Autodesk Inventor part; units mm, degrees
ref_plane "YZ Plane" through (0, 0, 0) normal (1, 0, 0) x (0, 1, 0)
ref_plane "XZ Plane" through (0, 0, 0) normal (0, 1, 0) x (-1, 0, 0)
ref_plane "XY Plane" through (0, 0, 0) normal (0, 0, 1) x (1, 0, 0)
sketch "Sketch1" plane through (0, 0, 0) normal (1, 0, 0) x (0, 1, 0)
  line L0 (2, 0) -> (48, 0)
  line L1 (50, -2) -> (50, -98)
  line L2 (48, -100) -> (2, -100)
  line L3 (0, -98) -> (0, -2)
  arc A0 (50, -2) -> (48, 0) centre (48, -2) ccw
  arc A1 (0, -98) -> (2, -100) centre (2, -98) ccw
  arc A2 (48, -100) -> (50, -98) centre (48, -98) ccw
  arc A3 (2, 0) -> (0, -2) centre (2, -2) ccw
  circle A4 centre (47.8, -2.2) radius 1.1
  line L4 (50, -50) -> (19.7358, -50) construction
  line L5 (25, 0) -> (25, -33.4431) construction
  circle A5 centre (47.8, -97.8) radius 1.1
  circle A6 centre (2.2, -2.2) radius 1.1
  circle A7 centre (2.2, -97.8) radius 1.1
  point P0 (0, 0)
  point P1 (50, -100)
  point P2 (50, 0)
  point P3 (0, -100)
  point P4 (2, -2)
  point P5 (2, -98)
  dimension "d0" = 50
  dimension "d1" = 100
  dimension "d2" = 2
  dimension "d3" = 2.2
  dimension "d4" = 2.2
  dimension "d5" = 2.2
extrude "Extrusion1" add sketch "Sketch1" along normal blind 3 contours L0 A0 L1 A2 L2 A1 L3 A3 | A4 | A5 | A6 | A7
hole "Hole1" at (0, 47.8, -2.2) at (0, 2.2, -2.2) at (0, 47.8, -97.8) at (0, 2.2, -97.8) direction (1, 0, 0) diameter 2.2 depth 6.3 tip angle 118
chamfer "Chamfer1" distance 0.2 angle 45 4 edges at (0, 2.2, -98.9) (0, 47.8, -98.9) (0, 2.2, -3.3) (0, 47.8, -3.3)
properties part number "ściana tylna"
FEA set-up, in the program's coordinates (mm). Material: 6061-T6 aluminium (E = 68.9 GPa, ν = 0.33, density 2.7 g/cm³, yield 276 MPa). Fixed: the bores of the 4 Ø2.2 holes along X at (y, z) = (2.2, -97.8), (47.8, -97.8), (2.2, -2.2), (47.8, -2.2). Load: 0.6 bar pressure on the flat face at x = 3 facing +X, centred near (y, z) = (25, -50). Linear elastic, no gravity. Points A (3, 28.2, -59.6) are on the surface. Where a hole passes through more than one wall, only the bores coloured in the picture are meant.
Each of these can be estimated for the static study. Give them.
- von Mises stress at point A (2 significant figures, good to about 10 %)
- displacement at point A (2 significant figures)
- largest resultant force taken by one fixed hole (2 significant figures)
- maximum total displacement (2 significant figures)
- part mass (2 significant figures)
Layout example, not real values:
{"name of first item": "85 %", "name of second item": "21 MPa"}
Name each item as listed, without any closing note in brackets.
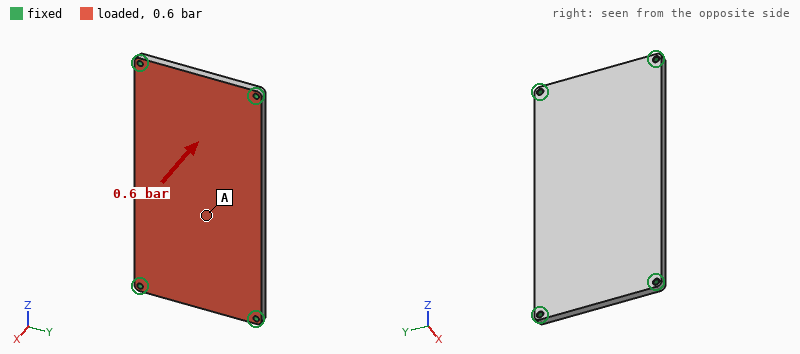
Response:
{"von Mises stress at point A": "16 MPa", "displacement at point A": "0.13 mm", "largest resultant force taken by one fixed hole": "75 N", "maximum total displacement": "0.14 mm", "part mass": "40 g"}
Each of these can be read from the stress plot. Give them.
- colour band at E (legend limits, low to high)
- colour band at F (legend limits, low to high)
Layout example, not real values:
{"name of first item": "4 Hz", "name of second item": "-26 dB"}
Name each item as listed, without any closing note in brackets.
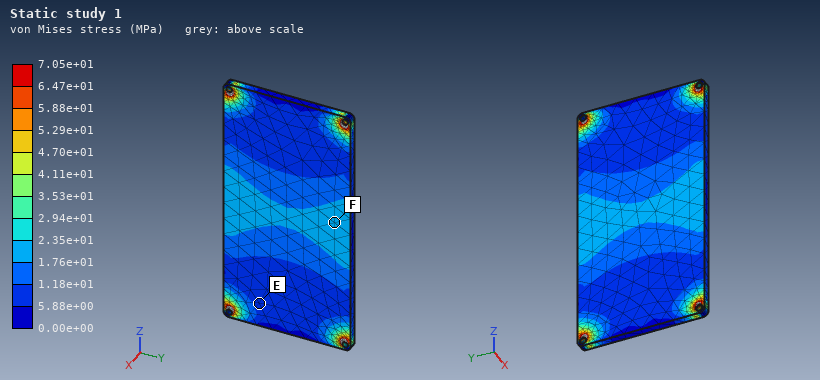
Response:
{"colour band at E": "5.88e+00 to 1.18e+01 MPa", "colour band at F": "1.76e+01 to 2.35e+01 MPa"}
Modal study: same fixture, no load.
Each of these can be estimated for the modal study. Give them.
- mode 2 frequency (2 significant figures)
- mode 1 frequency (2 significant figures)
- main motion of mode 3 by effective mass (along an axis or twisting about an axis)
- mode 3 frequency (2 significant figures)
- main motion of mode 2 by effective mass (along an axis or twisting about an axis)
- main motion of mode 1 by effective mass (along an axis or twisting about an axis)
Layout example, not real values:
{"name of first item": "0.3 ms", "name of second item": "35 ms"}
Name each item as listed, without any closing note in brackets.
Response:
{"mode 2 frequency": "2600 Hz", "mode 1 frequency": "1300 Hz", "main motion of mode 3 by effective mass": "twisting about Y", "mode 3 frequency": "3700 Hz", "main motion of mode 2 by effective mass": "twisting about Z", "main motion of mode 1 by effective mass": "along X"}
